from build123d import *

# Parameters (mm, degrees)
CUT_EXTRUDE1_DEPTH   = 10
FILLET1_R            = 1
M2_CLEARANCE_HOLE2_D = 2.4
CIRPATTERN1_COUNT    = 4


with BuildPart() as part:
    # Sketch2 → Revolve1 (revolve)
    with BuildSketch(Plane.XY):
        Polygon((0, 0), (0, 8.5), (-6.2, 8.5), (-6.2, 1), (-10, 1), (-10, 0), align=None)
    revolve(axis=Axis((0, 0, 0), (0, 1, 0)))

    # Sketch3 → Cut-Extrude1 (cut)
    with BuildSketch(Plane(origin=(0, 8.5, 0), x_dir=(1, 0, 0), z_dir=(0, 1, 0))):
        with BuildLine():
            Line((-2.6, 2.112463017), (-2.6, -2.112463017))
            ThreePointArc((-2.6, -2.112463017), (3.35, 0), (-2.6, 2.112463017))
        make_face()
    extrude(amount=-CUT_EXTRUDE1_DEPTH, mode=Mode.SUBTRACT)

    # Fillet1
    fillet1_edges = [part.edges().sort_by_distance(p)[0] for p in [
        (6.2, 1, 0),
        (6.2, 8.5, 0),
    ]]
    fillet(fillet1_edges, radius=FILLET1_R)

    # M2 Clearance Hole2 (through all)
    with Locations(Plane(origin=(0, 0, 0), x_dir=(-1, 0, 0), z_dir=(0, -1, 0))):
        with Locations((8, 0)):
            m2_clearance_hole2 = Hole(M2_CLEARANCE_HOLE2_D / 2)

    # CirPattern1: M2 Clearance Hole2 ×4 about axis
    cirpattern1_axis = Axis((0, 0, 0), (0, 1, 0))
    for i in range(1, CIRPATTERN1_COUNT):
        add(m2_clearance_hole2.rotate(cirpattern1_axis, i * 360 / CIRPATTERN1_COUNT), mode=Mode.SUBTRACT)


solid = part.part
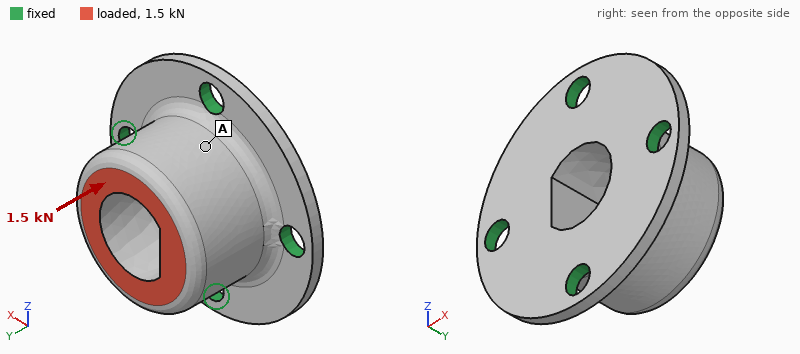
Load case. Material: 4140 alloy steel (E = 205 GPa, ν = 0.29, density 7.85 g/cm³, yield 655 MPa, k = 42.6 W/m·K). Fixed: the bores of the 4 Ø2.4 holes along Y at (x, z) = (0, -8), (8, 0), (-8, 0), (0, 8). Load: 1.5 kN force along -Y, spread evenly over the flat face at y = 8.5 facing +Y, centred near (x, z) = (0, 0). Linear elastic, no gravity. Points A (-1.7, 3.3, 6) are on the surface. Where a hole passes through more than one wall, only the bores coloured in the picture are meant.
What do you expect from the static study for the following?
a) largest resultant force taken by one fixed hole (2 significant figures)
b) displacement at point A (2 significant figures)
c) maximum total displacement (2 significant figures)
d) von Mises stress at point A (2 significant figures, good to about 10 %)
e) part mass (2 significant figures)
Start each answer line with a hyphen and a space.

- 440 N
- 2.5 µm
- 3.2 µm
- 33 MPa
- 7.2 g
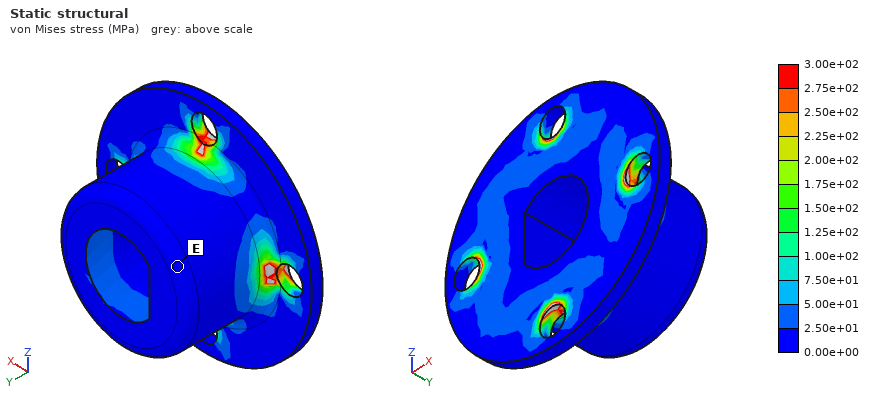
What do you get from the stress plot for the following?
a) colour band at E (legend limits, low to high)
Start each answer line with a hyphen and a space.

- 0.00e+00 to 2.50e+01 MPa
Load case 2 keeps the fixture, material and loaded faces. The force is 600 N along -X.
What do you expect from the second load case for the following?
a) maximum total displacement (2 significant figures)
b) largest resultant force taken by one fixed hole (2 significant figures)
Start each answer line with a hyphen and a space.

- 4.7 µm
- 420 N
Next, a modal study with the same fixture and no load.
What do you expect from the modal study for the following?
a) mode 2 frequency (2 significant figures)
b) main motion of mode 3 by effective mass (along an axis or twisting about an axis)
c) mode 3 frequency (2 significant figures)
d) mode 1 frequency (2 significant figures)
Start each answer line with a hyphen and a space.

- 39 kHz
- along Y
- 47 kHz
- 39 kHz
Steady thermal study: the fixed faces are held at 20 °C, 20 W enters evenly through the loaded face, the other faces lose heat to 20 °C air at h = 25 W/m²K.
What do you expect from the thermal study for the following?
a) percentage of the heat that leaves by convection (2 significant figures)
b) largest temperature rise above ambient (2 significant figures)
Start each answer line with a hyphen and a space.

- 3.9 %
- 75 K
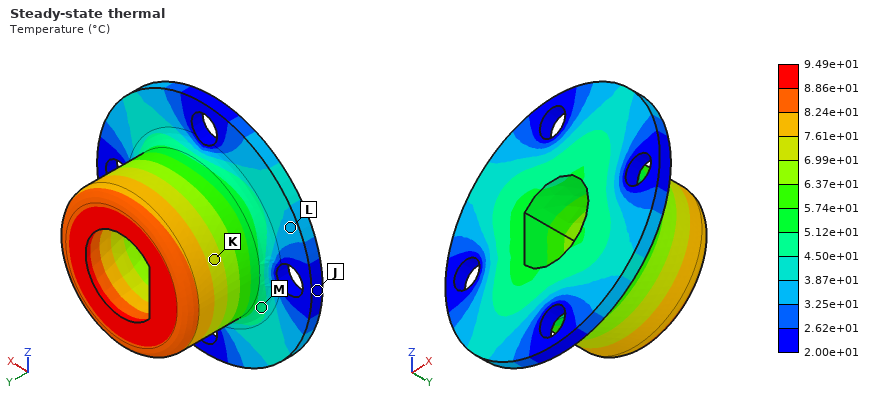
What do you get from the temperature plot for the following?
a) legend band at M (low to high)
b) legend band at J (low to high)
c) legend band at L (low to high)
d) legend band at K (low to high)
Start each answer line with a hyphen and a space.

- 4.50e+01 to 5.12e+01 °C
- 2.00e+01 to 2.62e+01 °C
- 3.25e+01 to 3.87e+01 °C
- 6.99e+01 to 7.61e+01 °C
